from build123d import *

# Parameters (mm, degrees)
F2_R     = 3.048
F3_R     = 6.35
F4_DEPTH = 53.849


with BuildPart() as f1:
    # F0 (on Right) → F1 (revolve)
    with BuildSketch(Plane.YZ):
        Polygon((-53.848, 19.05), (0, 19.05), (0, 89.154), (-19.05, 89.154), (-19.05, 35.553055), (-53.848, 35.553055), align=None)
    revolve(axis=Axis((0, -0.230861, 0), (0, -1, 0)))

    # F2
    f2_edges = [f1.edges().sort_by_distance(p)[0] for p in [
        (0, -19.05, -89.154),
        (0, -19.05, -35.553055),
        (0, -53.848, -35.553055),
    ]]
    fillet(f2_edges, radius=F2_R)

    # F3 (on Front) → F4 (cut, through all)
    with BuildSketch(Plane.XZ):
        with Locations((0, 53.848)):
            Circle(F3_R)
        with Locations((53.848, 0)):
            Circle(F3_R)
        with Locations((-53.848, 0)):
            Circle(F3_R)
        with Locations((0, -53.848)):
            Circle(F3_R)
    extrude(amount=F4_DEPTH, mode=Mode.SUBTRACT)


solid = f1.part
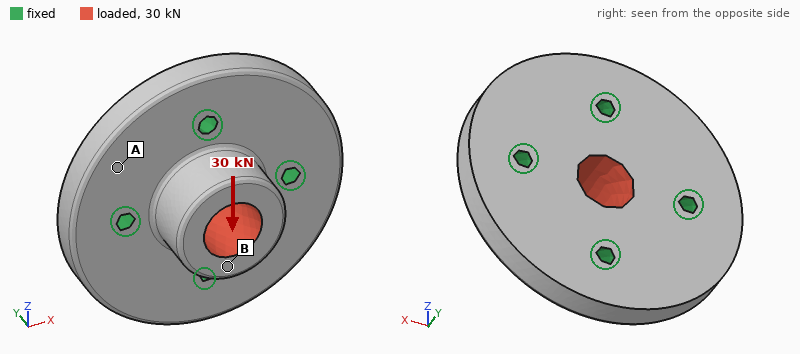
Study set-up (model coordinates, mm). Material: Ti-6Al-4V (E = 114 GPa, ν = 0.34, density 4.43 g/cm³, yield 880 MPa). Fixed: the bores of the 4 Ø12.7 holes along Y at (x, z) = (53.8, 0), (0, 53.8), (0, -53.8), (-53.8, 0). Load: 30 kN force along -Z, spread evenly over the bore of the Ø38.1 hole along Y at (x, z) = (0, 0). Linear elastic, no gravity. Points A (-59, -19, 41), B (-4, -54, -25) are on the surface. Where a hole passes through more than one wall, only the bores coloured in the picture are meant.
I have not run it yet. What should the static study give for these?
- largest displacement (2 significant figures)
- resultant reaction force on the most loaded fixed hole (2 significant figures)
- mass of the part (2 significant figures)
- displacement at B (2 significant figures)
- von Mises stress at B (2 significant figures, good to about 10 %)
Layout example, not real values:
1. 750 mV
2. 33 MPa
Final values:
1. 14 µm
2. 11 kN
3. 2.4 kg
4. 14 µm
5. 10 MPa
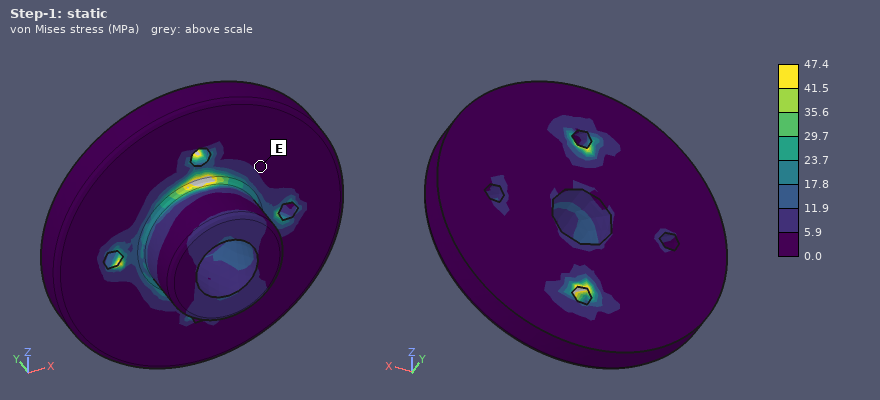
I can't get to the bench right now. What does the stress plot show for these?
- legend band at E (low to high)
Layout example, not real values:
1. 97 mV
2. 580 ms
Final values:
1. 0.0 to 5.9 MPa
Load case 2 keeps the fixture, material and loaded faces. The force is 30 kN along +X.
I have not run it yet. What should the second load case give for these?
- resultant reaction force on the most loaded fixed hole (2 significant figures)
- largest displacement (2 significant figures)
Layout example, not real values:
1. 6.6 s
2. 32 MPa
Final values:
1. 11 kN
2. 14 µm
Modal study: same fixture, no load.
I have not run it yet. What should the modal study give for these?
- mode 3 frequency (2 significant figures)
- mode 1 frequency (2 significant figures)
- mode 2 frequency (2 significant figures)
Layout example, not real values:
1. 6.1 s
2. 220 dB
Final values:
1. 6300 Hz
2. 5800 Hz
3. 6300 Hz
